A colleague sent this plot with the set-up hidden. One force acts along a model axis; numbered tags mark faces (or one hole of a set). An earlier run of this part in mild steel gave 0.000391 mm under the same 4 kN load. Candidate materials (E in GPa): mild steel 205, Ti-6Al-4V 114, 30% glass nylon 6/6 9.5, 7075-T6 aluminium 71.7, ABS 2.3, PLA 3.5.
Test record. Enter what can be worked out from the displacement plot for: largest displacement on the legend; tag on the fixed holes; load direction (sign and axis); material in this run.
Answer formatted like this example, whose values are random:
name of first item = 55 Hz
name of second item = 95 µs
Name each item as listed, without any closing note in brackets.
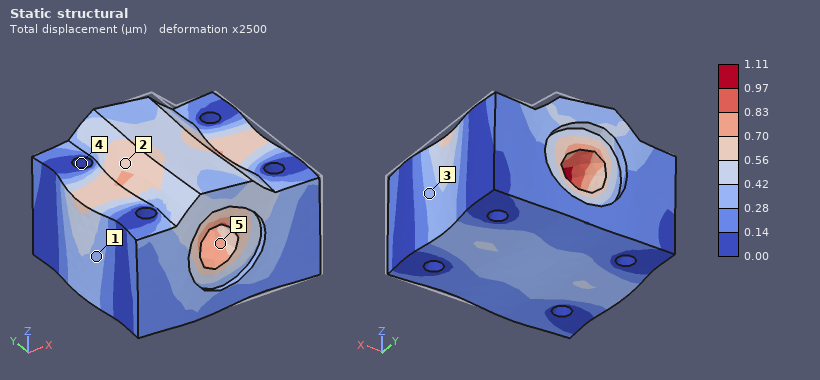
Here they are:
largest displacement on the legend = 1.11 µm
tag on the fixed holes = 4
load direction = -X
material in this run = 7075-T6 aluminium
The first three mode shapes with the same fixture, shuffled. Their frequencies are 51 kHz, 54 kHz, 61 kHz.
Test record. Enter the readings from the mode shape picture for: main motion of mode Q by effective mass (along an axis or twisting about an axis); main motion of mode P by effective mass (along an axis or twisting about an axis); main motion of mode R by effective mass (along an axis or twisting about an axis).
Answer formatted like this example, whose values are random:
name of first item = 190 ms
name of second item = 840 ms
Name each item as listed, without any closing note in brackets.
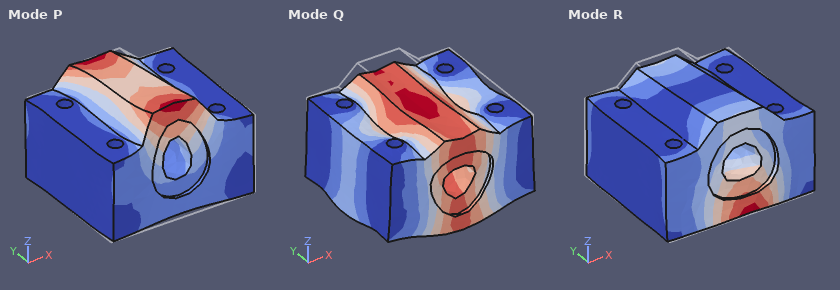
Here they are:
main motion of mode Q by effective mass = along Z
main motion of mode P by effective mass = along Y
main motion of mode R by effective mass = along Y
